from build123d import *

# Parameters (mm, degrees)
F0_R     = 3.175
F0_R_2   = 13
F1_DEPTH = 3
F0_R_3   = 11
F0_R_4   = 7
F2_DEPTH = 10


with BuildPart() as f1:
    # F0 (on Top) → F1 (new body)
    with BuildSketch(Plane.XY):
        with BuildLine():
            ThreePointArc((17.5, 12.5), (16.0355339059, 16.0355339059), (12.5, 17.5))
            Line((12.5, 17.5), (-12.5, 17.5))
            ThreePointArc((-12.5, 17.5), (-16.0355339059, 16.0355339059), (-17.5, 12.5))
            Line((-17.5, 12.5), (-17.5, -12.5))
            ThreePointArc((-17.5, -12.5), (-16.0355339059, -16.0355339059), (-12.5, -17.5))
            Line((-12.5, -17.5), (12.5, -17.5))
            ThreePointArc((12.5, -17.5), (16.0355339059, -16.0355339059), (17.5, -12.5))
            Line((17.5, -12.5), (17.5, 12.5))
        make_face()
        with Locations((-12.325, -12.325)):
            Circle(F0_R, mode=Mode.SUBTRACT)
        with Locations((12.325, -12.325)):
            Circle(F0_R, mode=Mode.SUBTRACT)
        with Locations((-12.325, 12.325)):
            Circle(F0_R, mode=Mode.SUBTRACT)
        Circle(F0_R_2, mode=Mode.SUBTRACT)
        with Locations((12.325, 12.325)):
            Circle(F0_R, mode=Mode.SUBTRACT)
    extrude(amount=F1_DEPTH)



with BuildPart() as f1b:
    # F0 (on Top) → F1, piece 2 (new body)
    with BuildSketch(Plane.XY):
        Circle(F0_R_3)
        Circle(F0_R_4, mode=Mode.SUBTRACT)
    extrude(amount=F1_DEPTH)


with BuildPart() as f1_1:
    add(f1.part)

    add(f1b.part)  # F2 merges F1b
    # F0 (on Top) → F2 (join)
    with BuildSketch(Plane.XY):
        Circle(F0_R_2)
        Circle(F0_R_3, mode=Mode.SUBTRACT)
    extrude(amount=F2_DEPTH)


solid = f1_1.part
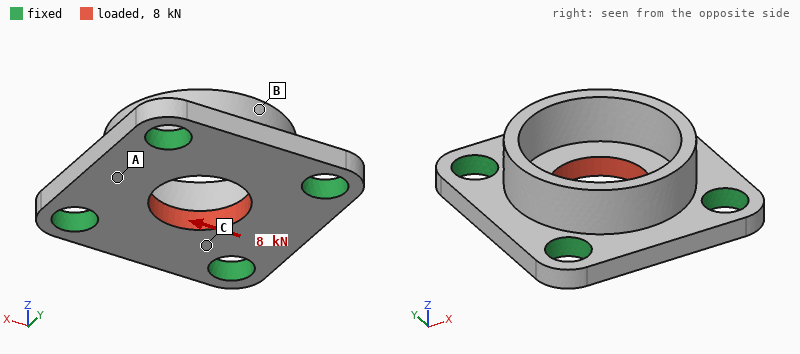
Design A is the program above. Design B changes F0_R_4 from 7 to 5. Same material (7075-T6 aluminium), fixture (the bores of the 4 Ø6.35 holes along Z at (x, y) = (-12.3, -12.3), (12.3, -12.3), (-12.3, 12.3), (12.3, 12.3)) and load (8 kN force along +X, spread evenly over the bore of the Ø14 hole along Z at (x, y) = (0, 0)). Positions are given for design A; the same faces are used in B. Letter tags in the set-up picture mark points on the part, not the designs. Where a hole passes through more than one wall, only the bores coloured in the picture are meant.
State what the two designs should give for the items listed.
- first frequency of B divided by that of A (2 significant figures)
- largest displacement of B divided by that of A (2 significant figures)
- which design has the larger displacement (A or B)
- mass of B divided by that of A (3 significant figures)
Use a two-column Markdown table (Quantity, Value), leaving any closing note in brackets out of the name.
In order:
| Quantity | Value |
|---|---|
| first frequency of B divided by that of A | 1.0 |
| largest displacement of B divided by that of A | 1.1 |
| which design has the larger displacement | B |
| mass of B divided by that of A | 1.06 |
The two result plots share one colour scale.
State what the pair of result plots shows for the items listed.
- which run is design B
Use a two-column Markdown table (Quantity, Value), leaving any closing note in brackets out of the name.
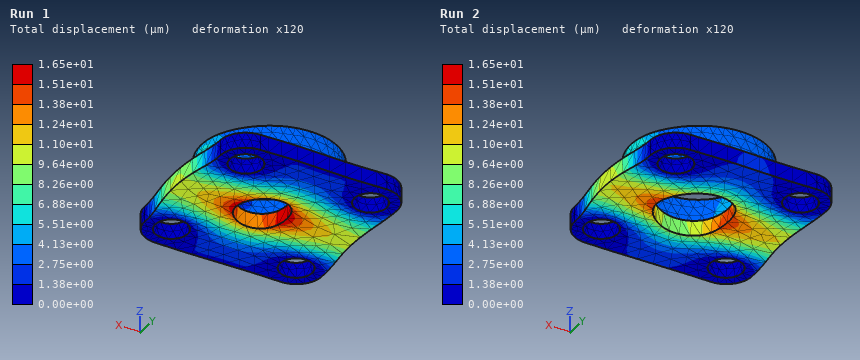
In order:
| Quantity | Value |
|---|---|
| which run is design B | Run 1 |
